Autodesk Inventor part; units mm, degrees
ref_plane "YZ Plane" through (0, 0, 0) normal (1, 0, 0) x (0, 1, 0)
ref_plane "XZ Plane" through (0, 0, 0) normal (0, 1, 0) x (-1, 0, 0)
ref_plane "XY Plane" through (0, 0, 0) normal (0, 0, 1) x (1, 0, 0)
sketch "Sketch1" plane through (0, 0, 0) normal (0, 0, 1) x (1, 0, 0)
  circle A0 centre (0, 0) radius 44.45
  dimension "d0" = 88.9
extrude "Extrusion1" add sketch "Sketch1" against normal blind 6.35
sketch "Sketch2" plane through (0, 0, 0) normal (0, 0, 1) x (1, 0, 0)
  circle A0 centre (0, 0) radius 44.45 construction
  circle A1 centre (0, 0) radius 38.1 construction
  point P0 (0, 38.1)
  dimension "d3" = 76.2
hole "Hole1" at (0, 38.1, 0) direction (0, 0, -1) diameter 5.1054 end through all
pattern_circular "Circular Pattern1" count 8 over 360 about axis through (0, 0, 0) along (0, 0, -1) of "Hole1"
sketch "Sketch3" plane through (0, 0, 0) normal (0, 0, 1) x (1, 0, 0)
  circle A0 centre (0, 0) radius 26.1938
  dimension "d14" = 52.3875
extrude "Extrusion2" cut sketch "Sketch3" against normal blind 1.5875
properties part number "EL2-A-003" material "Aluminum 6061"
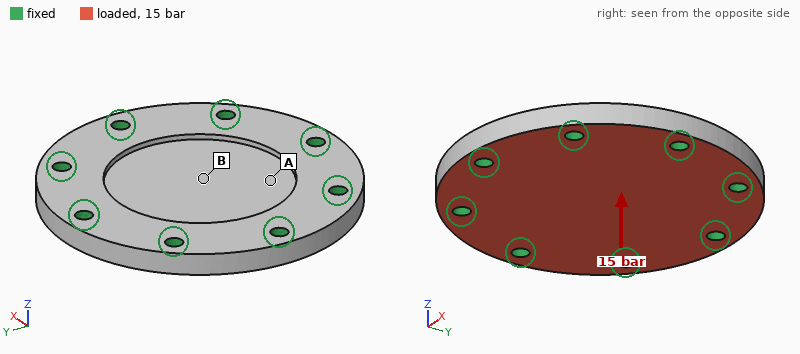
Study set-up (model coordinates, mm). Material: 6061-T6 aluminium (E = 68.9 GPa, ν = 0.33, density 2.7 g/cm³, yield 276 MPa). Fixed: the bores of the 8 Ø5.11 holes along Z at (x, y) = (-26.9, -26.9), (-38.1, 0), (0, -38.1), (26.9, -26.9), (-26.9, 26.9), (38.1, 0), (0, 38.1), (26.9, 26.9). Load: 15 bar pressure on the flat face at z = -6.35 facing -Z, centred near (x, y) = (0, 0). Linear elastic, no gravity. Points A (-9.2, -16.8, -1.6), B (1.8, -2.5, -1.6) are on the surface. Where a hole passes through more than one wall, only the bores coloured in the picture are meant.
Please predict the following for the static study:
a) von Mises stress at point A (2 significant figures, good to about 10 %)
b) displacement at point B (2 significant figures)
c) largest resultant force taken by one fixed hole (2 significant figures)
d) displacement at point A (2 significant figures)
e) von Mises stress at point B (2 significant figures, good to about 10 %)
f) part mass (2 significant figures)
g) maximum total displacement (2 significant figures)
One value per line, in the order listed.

16 MPa
54 µm
1.2 kN
30 µm
35 MPa
94 g
54 µm
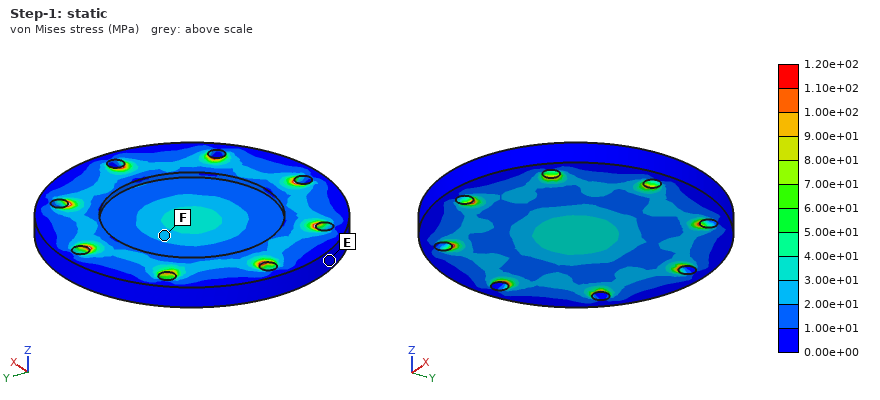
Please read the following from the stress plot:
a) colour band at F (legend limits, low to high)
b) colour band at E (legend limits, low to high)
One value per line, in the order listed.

2.00e+01 to 3.00e+01 MPa
0.00e+00 to 1.00e+01 MPa
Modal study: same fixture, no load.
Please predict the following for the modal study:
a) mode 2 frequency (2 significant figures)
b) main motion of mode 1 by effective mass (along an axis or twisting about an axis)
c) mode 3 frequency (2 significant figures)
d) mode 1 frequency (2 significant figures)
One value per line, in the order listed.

17 kHz
along Z
17 kHz
9200 Hz
